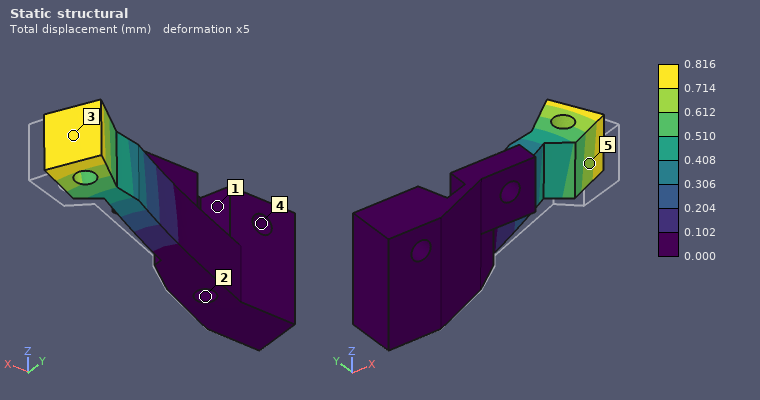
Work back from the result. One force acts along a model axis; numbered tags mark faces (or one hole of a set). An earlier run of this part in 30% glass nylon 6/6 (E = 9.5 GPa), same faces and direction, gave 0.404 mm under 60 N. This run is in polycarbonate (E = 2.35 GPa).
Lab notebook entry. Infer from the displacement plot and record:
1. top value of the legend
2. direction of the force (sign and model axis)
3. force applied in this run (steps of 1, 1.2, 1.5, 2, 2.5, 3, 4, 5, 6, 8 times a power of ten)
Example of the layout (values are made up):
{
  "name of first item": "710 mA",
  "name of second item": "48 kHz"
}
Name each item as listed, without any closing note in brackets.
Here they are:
{
  "top value of the legend": "0.816 mm",
  "direction of the force": "+Y",
  "force applied in this run": "30 N"
}
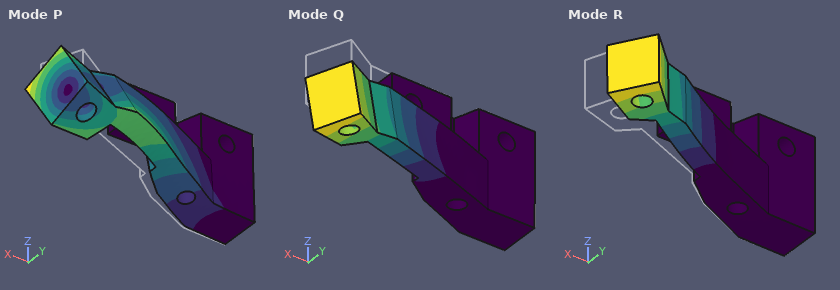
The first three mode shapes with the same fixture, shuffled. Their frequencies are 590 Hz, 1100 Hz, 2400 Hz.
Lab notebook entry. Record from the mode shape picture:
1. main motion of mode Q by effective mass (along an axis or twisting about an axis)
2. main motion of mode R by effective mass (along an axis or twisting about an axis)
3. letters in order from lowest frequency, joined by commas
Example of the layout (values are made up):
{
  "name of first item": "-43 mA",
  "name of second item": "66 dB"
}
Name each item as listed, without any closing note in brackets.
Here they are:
{
  "main motion of mode Q by effective mass": "along Z",
  "main motion of mode R by effective mass": "along Y",
  "letters in order from lowest frequency, joined by commas": "R, Q, P"
}
